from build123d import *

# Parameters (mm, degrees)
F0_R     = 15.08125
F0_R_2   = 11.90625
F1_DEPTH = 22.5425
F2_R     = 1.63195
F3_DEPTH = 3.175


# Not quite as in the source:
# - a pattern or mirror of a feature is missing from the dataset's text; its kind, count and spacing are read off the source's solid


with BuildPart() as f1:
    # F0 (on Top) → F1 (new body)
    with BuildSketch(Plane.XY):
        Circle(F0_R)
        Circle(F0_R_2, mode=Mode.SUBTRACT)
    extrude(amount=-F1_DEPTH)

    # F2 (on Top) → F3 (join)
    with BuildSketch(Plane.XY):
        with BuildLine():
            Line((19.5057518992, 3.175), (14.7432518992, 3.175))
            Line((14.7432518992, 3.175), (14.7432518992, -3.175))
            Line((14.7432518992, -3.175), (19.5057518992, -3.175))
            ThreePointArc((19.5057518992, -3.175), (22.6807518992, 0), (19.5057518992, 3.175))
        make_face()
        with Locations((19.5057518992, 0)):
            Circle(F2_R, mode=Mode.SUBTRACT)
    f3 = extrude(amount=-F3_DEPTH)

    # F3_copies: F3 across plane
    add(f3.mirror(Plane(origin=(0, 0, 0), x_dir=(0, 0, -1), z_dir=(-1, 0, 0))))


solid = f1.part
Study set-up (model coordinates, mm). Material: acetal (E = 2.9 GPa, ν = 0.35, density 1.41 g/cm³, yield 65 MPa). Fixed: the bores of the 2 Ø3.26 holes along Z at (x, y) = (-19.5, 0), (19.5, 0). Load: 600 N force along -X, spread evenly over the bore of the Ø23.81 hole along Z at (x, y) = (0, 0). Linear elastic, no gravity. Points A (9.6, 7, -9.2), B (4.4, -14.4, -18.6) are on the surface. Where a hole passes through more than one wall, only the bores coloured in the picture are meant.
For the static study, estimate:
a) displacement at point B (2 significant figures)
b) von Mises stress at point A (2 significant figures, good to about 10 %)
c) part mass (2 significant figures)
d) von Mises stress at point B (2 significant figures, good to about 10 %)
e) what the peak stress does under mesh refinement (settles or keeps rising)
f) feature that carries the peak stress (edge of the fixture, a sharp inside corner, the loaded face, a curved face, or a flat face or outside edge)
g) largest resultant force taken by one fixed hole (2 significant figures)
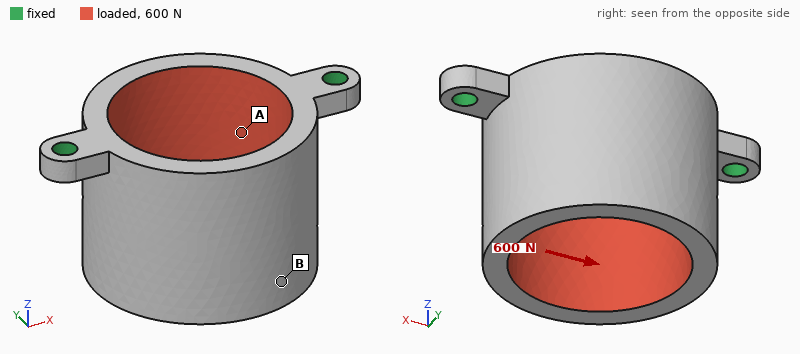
0.20 mm
10 MPa
8.9 g
3.0 MPa
keeps rising
edge of the fixture
350 N
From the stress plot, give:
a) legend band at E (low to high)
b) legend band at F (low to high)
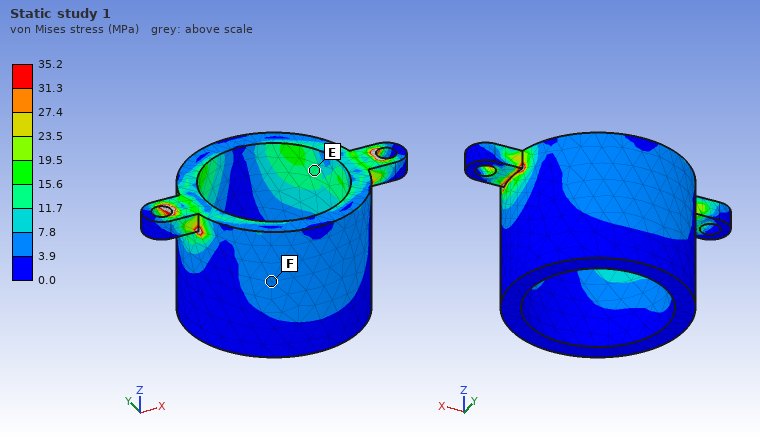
11.7 to 15.6 MPa
3.9 to 7.8 MPa
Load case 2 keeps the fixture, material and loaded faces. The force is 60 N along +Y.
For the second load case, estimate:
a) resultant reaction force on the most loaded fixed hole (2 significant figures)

30 N
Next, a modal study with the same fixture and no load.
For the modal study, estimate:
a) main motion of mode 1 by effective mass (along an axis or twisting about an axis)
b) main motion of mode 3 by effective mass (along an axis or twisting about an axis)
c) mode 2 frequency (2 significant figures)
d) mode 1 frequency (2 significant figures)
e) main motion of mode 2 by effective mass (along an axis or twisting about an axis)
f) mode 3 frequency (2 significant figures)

along Y
along X
2600 Hz
580 Hz
along Z
3100 Hz
